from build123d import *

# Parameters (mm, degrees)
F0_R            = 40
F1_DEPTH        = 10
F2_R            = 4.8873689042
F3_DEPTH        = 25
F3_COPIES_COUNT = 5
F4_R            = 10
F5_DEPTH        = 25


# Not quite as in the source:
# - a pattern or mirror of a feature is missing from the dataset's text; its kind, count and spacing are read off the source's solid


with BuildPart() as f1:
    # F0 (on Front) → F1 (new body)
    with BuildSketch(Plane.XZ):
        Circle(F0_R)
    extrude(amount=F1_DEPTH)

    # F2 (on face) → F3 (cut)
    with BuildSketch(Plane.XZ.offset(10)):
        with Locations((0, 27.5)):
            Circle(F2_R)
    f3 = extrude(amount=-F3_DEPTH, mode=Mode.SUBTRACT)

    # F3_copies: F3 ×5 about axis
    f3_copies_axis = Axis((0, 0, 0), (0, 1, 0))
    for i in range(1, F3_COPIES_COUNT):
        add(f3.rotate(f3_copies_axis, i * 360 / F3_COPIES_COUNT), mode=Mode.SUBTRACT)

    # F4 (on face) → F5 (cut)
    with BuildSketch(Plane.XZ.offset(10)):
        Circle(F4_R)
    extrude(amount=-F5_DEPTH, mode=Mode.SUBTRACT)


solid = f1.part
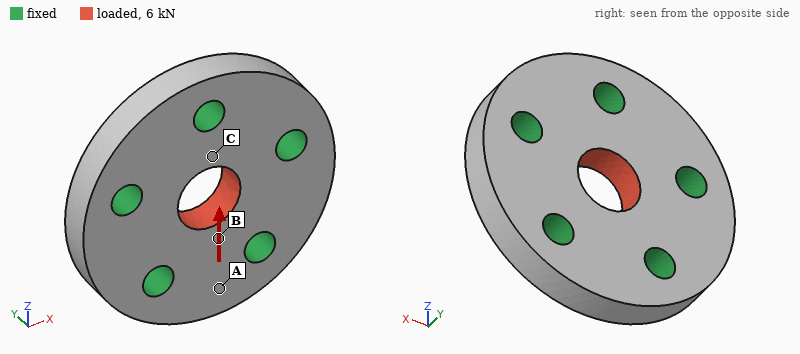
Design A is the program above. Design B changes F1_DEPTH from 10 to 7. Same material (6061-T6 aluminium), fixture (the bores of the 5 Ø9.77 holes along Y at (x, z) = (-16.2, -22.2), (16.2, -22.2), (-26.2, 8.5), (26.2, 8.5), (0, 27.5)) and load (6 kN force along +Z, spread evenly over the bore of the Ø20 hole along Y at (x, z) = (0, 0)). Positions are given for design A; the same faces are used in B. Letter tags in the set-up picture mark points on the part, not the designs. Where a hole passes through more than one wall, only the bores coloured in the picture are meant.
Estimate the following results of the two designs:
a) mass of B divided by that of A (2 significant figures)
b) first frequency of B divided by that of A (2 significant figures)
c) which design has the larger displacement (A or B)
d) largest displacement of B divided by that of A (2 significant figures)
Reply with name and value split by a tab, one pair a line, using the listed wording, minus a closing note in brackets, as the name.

mass of B divided by that of A	0.70
first frequency of B divided by that of A	0.81
which design has the larger displacement	B
largest displacement of B divided by that of A	1.4
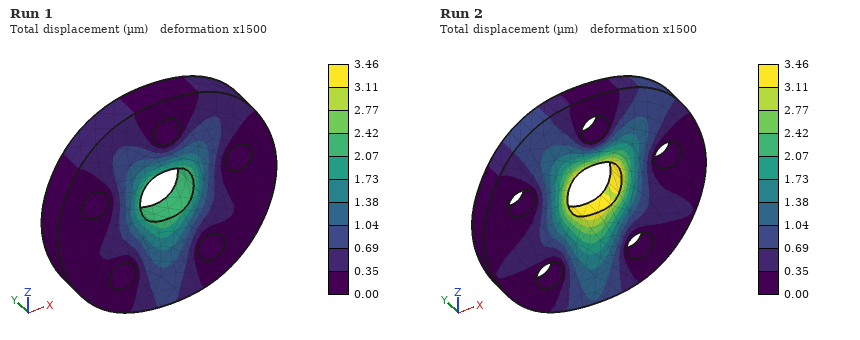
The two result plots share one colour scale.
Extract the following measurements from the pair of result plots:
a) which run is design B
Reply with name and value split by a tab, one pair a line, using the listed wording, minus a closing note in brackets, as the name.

which run is design B	Run 2
